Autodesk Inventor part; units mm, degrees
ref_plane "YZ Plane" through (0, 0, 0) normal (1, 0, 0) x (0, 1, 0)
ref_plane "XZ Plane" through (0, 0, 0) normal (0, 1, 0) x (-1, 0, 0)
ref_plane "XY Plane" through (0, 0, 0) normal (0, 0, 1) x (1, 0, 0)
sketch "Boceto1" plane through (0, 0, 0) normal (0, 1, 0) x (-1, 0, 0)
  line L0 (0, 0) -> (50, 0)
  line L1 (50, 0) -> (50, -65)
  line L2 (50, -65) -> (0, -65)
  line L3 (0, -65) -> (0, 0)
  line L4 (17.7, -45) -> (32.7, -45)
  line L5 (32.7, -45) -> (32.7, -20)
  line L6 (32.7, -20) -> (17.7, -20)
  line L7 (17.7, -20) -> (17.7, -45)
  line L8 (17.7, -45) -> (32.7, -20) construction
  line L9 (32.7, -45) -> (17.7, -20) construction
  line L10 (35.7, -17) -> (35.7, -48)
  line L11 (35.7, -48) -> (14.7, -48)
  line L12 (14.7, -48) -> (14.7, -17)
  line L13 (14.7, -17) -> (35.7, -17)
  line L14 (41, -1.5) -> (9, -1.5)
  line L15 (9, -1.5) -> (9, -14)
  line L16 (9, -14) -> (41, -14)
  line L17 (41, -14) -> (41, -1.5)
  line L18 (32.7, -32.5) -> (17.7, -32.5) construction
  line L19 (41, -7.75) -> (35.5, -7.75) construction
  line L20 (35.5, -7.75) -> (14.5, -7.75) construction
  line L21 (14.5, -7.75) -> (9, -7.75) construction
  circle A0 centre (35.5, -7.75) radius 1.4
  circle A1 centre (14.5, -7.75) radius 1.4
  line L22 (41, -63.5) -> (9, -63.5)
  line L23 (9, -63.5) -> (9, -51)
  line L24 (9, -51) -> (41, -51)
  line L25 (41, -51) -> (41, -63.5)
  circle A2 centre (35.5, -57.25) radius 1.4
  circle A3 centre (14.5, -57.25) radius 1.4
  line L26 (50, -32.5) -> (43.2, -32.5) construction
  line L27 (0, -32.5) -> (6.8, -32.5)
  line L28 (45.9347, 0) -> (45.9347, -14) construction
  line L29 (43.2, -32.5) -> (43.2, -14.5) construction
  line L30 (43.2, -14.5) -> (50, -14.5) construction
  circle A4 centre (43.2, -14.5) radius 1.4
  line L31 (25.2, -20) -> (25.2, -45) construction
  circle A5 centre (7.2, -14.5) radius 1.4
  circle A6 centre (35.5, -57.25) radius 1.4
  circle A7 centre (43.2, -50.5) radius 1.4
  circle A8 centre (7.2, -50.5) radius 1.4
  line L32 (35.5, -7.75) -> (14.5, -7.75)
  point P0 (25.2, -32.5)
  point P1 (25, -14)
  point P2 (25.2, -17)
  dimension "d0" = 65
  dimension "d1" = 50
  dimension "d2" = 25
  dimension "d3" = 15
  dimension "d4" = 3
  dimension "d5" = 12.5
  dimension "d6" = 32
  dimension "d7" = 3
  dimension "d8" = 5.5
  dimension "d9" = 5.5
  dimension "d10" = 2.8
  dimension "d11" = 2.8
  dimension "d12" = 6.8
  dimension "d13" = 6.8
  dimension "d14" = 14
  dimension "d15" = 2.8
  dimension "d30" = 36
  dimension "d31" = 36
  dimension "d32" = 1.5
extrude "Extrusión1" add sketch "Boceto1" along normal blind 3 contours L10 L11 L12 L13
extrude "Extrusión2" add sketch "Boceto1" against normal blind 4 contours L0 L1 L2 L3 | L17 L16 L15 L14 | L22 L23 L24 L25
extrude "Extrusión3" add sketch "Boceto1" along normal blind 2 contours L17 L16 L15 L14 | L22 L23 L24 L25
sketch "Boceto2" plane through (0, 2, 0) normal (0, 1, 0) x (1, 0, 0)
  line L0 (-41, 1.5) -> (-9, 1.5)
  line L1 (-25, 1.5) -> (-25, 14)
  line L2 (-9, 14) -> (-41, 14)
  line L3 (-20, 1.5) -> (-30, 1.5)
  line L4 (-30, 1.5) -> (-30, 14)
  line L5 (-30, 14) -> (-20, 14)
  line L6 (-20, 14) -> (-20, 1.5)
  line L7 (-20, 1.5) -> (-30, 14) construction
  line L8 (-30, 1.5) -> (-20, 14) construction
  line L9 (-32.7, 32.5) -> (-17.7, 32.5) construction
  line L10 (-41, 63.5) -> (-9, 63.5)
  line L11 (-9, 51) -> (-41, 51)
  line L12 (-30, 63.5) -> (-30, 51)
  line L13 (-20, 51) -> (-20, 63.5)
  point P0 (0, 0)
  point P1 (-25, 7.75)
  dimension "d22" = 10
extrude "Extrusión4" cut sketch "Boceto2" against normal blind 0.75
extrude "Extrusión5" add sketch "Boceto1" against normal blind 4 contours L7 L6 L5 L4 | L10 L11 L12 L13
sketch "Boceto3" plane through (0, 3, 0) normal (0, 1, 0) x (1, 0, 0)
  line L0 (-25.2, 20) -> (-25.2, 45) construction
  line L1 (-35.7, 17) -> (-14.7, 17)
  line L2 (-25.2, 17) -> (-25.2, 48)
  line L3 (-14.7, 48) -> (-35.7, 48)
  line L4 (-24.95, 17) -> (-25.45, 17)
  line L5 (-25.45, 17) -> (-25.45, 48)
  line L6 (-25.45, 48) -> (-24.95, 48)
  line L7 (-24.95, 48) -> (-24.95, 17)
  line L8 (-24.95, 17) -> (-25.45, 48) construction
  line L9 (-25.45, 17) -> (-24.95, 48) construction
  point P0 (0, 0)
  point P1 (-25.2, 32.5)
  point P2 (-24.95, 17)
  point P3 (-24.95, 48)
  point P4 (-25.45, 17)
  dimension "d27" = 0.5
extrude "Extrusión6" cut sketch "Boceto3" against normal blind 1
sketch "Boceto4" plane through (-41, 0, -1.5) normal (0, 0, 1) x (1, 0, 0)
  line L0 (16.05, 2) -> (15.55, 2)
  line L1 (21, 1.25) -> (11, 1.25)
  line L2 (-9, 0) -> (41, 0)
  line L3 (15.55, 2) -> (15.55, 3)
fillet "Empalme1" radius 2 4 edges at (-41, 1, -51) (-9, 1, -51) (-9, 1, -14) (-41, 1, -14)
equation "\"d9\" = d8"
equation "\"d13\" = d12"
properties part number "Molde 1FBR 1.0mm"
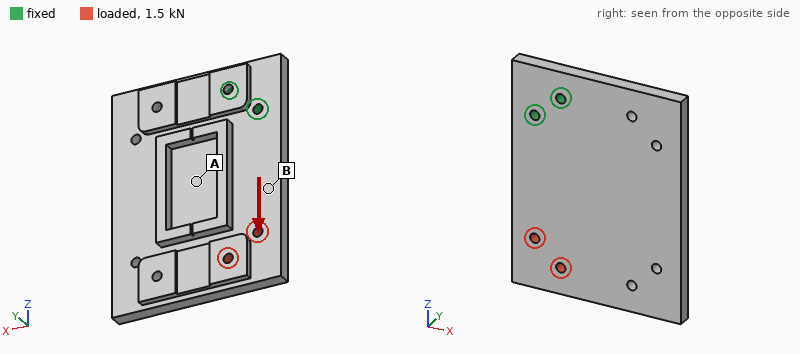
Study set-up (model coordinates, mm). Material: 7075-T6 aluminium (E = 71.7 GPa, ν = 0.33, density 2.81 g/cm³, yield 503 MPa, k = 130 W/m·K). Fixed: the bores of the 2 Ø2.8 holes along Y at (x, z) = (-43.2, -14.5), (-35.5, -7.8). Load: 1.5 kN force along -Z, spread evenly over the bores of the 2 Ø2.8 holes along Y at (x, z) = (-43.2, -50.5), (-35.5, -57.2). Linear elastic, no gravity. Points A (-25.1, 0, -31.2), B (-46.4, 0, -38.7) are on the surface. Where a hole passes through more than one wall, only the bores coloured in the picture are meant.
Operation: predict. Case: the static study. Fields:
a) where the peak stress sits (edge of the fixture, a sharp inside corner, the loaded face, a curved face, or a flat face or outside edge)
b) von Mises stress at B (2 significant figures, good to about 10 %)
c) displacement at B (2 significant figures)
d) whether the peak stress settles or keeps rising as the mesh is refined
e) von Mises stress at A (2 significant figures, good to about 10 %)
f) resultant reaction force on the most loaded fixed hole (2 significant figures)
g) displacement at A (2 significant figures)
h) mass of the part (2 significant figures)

edge of the fixture
20 MPa
13 µm
keeps rising
7.9 MPa
780 N
11 µm
42 g
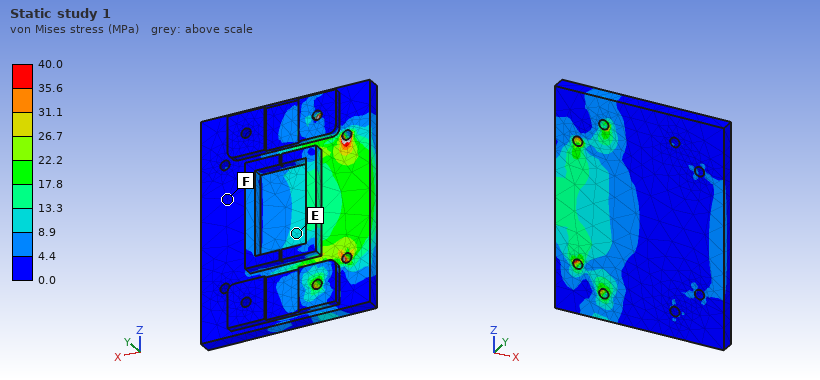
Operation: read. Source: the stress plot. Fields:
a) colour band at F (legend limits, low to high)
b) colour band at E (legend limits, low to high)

0.0 to 4.4 MPa
8.9 to 13.3 MPa
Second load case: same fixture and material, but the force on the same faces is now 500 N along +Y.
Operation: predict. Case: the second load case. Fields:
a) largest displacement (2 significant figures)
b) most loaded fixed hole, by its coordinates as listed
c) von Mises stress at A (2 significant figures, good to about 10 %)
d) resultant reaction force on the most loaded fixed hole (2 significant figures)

0.91 mm
(-43.2, -14.5)
43 MPa
1.1 kN
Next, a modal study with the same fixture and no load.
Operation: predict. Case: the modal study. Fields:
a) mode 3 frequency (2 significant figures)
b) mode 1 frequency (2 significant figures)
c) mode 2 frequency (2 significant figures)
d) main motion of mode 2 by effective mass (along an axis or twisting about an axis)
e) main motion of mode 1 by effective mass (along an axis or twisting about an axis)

3300 Hz
940 Hz
2300 Hz
twisting about Z
along Y
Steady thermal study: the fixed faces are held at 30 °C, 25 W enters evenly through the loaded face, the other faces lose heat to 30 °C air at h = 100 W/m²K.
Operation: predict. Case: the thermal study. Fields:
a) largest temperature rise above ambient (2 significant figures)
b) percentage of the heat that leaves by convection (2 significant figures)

39 K
51 %
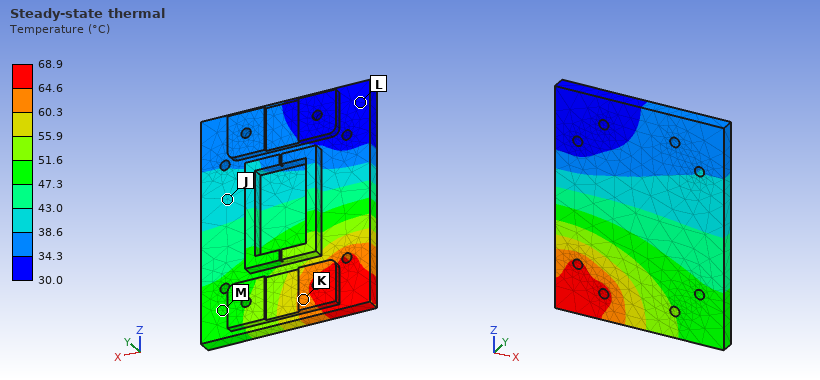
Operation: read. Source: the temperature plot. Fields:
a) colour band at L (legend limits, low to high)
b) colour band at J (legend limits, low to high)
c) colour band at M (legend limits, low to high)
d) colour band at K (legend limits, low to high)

30.0 to 34.3 °C
38.6 to 43.0 °C
47.3 to 51.6 °C
60.3 to 64.6 °C
